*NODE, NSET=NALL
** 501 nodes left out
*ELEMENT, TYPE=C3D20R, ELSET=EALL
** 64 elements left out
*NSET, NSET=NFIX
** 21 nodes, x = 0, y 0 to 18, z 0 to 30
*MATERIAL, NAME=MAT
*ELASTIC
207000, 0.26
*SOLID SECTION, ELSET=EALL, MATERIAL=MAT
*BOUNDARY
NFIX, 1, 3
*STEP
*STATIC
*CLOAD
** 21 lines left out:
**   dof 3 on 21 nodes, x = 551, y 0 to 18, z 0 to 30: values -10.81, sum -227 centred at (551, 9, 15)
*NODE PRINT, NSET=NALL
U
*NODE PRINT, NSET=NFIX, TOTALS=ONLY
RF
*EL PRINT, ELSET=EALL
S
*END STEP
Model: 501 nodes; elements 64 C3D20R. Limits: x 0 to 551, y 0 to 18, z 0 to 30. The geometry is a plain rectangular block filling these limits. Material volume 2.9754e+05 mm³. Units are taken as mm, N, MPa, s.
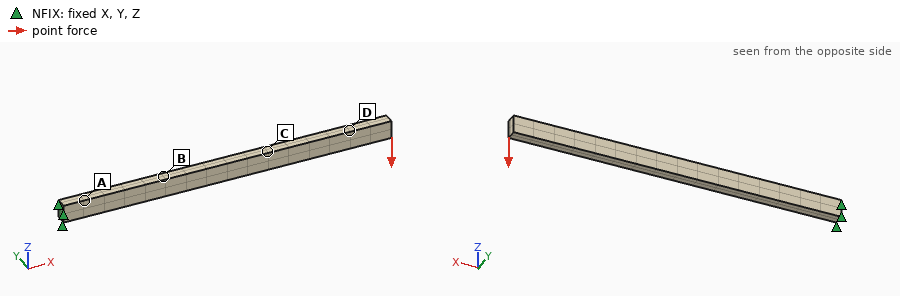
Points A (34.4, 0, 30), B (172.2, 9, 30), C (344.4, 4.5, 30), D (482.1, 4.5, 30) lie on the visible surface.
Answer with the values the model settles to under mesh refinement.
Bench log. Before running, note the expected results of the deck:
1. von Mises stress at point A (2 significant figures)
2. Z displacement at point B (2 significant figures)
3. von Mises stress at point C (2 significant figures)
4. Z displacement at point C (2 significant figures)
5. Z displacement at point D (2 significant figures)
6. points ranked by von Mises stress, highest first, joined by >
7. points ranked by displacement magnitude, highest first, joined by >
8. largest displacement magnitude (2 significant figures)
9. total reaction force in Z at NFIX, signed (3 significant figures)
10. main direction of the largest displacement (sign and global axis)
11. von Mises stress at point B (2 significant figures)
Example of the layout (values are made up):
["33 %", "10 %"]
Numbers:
["43 MPa", "-0.20 mm", "17 MPa", "-0.70 mm", "-1.2 mm", "A > B > C > D", "D > C > B > A", "1.5 mm", "227 N", "-Z", "32 MPa"]
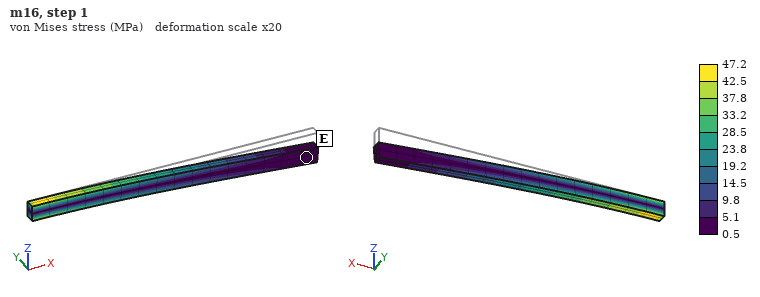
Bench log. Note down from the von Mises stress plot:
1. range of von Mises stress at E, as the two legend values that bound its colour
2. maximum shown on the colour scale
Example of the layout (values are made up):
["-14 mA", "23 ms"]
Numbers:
["0.5 to 5.1 MPa", "47.2 MPa"]
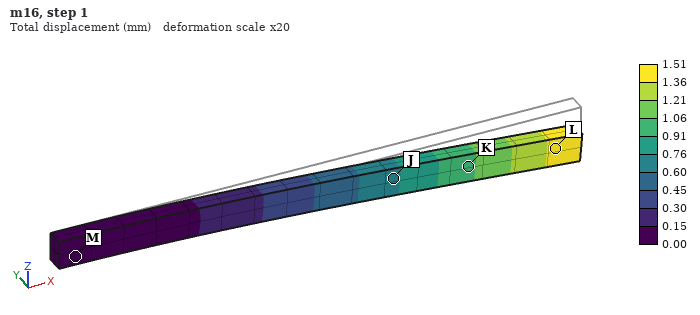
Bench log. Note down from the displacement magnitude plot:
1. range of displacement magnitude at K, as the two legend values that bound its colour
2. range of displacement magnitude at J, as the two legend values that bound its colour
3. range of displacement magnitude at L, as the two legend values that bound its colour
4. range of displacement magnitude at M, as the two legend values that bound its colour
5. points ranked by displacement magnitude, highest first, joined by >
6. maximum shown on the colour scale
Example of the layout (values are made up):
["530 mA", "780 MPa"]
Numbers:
["0.91 to 1.06 mm", "0.60 to 0.76 mm", "1.36 to 1.51 mm", "0.00 to 0.15 mm", "L > K > J > M", "1.51 mm"]
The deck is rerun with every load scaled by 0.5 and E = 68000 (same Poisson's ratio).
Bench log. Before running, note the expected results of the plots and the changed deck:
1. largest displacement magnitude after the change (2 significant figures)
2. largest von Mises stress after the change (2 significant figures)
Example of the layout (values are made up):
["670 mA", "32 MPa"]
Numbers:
["2.3 mm", "24 MPa"]
